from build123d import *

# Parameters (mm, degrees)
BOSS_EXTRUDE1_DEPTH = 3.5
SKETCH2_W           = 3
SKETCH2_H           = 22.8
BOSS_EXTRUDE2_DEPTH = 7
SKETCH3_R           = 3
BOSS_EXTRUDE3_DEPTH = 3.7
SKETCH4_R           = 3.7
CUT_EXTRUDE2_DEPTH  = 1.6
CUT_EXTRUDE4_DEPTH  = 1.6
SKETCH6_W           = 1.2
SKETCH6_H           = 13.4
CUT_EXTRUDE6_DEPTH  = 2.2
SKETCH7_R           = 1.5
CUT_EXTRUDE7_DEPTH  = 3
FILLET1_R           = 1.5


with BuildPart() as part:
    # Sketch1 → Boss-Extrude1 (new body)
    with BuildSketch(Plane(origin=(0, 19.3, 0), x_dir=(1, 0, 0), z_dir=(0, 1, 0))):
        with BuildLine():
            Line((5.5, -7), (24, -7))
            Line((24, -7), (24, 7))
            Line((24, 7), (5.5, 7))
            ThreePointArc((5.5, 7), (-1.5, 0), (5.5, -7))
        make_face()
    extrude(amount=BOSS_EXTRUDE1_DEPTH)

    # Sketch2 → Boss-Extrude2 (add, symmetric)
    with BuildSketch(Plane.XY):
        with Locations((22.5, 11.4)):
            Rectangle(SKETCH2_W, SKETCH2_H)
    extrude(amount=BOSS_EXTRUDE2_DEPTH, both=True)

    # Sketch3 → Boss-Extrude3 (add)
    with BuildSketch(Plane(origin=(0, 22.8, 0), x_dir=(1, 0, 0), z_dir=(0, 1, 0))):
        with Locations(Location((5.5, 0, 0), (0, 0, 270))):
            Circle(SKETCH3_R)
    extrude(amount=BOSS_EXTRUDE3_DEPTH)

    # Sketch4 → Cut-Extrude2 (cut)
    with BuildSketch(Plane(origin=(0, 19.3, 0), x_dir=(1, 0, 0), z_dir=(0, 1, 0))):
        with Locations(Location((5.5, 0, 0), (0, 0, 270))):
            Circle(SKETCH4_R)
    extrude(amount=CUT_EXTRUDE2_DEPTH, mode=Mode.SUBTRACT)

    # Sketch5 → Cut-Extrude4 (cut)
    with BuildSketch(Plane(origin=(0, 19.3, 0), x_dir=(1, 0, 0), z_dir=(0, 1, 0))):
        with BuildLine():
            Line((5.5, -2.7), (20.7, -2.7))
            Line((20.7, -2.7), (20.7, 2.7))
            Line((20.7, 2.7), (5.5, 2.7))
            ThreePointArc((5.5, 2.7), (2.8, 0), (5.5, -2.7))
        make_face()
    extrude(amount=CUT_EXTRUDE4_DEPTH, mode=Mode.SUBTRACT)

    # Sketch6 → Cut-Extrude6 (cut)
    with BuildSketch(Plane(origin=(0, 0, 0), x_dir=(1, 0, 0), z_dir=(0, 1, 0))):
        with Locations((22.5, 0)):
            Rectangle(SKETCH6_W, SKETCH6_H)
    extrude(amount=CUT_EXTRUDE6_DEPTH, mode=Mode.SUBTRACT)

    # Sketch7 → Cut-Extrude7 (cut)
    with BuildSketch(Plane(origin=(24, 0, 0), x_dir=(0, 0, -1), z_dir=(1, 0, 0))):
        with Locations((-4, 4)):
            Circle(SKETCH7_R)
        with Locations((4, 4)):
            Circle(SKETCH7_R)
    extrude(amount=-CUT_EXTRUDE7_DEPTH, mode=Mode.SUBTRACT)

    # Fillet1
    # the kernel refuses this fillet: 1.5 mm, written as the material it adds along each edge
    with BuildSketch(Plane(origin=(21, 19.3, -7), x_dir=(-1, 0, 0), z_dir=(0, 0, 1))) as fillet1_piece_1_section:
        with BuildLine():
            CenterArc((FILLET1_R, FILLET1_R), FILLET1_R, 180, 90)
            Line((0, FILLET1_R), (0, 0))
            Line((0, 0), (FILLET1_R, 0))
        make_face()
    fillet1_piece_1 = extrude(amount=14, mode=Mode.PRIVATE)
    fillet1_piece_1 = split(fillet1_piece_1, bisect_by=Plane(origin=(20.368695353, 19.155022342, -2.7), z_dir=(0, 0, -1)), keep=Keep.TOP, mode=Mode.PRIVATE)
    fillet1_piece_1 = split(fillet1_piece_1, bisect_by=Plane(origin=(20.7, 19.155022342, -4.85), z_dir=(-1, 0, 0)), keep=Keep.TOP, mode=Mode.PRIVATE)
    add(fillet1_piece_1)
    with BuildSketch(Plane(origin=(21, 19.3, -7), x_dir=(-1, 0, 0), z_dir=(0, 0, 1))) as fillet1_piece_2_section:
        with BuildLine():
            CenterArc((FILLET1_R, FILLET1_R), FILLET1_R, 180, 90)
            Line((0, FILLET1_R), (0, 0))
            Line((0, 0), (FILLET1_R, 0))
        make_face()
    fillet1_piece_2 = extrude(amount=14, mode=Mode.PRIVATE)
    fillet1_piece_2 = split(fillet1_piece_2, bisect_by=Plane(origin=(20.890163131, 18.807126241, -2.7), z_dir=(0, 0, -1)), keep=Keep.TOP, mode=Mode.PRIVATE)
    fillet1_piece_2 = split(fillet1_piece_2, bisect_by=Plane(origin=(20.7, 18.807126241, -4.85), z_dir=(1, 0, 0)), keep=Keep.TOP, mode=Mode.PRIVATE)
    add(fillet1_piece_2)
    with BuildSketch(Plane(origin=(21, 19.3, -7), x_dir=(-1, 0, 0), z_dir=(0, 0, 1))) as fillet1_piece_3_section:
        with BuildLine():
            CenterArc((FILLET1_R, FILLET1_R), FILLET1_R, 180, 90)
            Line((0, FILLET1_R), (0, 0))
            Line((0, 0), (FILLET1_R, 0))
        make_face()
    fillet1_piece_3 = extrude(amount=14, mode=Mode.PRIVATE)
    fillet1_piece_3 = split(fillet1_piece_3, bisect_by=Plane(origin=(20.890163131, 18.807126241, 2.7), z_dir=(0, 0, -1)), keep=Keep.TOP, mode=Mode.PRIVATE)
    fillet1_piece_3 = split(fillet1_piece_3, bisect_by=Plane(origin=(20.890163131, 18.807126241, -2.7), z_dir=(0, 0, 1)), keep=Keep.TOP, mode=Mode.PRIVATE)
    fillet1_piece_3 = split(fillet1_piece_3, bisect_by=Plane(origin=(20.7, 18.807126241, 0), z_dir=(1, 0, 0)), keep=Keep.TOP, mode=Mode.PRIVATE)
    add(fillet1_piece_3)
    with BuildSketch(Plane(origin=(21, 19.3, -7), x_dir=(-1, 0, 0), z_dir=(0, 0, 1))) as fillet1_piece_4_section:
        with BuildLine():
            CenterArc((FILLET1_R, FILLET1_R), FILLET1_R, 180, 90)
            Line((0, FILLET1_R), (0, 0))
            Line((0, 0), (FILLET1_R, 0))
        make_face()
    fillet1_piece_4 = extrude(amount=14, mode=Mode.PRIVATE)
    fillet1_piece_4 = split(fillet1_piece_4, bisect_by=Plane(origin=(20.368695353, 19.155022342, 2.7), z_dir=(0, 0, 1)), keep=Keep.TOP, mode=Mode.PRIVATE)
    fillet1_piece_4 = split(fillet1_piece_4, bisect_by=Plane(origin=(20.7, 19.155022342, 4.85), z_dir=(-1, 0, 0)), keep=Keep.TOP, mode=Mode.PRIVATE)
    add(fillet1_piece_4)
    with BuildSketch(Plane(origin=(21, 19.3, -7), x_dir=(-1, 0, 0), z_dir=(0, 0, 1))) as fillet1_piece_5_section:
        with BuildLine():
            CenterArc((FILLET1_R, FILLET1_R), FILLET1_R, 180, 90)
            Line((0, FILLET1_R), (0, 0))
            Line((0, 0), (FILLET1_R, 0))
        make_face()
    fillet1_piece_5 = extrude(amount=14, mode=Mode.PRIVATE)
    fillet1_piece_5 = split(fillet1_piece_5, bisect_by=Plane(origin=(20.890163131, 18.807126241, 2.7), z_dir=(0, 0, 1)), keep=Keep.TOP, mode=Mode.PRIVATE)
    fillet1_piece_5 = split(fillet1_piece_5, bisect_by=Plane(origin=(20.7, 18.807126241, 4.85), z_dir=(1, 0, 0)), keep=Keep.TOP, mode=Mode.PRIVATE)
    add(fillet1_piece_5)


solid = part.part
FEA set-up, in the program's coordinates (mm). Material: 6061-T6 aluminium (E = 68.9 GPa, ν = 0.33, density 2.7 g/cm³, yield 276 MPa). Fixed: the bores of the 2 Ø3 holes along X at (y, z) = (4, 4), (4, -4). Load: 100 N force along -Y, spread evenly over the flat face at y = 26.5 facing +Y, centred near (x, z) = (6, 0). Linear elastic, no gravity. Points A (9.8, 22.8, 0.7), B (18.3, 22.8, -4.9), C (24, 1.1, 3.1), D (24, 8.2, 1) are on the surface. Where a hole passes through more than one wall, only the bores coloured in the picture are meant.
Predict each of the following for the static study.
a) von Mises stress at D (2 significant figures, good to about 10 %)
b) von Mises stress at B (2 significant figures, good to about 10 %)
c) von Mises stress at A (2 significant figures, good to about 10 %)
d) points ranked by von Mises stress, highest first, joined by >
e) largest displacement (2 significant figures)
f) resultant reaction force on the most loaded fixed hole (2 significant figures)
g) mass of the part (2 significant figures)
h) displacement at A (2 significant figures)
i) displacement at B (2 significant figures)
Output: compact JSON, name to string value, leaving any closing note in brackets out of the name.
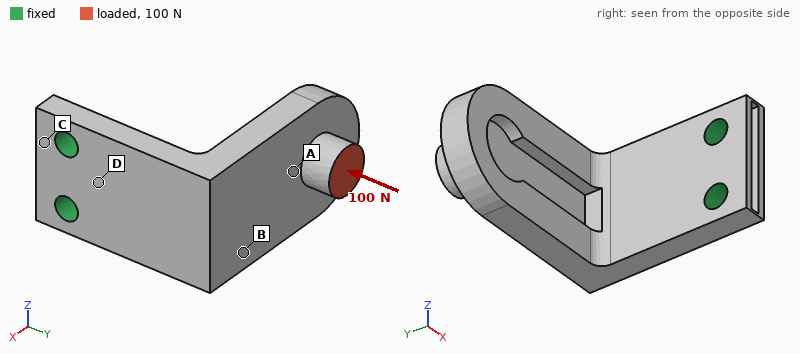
{"von Mises stress at D": "69 MPa", "von Mises stress at B": "55 MPa", "von Mises stress at A": "19 MPa", "points ranked by von Mises stress, highest first, joined by >": "D > B > A > C", "largest displacement": "0.39 mm", "resultant reaction force on the most loaded fixed hole": "51 N", "mass of the part": "5.0 g", "displacement at A": "0.22 mm", "displacement at B": "0.13 mm"}
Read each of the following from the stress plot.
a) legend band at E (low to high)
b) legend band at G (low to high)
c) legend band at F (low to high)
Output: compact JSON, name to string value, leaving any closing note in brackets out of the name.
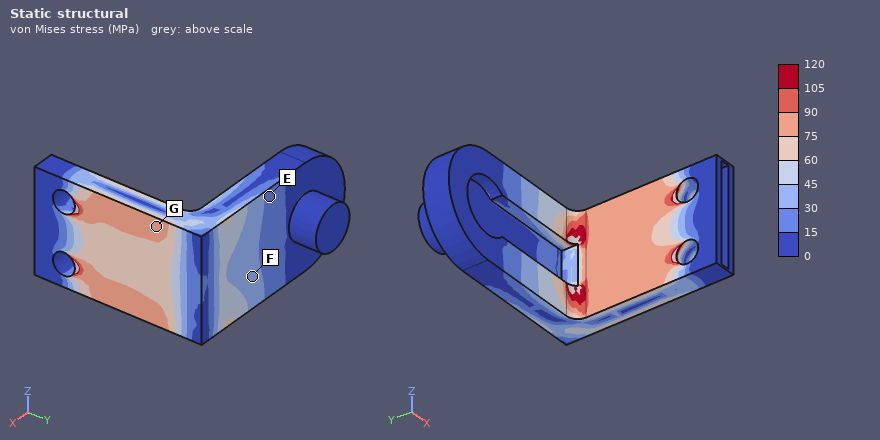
{"legend band at E": "15 to 30 MPa", "legend band at G": "75 to 90 MPa", "legend band at F": "30 to 45 MPa"}
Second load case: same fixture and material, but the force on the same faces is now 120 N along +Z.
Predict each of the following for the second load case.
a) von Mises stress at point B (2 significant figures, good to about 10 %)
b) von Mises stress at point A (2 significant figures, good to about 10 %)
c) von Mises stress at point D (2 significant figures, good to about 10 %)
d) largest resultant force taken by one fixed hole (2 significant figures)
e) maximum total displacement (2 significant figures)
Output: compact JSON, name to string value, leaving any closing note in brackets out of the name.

{"von Mises stress at point B": "19 MPa", "von Mises stress at point A": "28 MPa", "von Mises stress at point D": "50 MPa", "largest resultant force taken by one fixed hole": "340 N", "maximum total displacement": "0.19 mm"}
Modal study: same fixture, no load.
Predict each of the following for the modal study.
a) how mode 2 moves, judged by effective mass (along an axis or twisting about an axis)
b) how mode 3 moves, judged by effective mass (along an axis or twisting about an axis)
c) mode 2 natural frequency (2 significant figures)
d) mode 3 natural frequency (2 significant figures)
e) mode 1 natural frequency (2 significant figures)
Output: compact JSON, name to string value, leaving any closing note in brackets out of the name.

{"how mode 2 moves, judged by effective mass": "along Z", "how mode 3 moves, judged by effective mass": "along X", "mode 2 natural frequency": "3300 Hz", "mode 3 natural frequency": "6400 Hz", "mode 1 natural frequency": "2000 Hz"}
